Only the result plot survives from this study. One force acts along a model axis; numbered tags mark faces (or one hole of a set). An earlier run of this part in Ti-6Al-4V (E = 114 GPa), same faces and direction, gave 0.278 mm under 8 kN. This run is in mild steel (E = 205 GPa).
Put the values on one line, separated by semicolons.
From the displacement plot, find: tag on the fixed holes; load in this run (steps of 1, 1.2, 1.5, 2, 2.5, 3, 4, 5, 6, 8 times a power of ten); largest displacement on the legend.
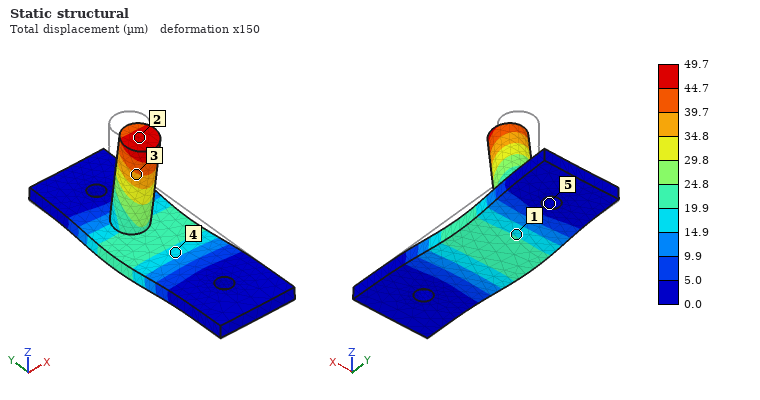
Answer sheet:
5; 2.5 kN; 49.7 µm
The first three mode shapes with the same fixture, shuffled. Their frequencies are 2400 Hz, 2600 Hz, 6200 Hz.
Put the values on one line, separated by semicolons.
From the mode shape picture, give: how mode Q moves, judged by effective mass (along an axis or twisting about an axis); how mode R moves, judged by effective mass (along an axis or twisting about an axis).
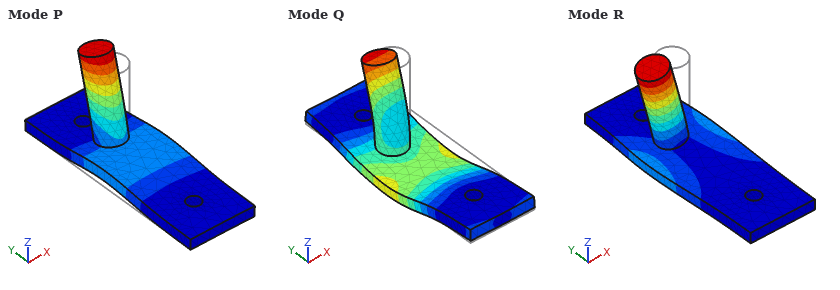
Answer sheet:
along Z; along X
